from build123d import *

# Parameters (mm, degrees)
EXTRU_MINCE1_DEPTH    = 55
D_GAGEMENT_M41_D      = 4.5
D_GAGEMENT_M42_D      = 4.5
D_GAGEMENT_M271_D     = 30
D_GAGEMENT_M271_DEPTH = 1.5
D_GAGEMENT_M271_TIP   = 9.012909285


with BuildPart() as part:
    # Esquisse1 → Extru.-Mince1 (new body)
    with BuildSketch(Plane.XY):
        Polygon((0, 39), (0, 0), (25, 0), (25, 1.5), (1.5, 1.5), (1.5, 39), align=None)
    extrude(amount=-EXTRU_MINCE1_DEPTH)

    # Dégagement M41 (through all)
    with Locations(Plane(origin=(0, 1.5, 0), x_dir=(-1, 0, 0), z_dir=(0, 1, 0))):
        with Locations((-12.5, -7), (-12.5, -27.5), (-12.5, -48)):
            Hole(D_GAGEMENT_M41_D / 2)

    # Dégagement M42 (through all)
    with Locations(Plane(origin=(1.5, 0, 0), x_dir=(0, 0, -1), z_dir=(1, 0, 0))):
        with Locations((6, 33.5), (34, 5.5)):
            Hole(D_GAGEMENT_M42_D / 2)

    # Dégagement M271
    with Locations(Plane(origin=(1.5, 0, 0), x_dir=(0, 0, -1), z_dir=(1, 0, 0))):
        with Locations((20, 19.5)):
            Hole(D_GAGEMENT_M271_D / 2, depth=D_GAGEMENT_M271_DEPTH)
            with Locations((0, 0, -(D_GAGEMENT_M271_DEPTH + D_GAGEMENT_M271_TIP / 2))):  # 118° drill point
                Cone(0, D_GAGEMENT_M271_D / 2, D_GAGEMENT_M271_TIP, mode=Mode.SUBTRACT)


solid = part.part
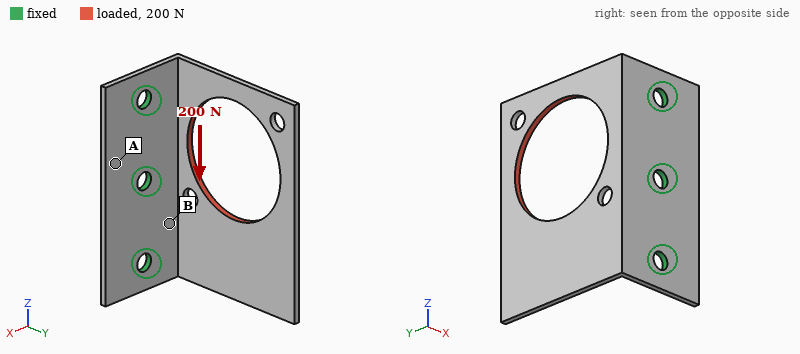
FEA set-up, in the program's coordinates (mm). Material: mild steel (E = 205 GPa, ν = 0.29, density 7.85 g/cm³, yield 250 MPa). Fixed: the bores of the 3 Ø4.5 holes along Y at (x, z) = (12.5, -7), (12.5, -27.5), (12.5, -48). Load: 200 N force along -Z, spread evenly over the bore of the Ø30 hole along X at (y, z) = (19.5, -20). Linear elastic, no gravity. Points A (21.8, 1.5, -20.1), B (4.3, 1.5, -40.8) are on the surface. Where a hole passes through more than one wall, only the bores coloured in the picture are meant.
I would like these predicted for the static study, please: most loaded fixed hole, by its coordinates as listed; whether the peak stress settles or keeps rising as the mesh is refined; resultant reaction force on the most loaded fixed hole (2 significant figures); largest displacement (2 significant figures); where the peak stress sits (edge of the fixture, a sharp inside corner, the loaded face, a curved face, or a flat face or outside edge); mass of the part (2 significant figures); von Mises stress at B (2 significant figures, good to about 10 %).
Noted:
(12.5, -7)
keeps rising
130 N
99 µm
edge of the fixture
31 g
43 MPa
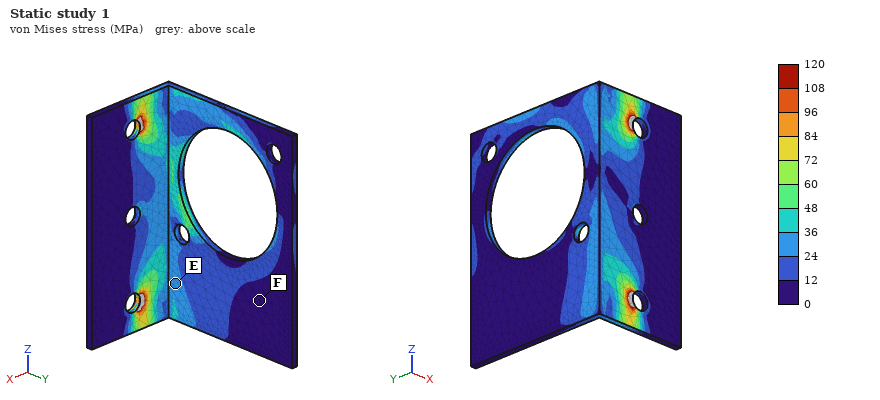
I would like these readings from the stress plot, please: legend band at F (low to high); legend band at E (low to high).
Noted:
0 to 12 MPa
24 to 36 MPa
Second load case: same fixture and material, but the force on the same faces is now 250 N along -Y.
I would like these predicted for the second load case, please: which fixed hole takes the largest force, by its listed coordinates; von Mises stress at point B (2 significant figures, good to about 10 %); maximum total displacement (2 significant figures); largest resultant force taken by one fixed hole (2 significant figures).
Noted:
(12.5, -7)
33 MPa
0.20 mm
130 N
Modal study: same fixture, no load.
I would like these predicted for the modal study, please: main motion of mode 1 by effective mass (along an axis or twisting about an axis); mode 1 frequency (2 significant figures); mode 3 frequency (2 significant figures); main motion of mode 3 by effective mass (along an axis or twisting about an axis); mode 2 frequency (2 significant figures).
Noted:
along X
580 Hz
2500 Hz
along Z
1200 Hz
